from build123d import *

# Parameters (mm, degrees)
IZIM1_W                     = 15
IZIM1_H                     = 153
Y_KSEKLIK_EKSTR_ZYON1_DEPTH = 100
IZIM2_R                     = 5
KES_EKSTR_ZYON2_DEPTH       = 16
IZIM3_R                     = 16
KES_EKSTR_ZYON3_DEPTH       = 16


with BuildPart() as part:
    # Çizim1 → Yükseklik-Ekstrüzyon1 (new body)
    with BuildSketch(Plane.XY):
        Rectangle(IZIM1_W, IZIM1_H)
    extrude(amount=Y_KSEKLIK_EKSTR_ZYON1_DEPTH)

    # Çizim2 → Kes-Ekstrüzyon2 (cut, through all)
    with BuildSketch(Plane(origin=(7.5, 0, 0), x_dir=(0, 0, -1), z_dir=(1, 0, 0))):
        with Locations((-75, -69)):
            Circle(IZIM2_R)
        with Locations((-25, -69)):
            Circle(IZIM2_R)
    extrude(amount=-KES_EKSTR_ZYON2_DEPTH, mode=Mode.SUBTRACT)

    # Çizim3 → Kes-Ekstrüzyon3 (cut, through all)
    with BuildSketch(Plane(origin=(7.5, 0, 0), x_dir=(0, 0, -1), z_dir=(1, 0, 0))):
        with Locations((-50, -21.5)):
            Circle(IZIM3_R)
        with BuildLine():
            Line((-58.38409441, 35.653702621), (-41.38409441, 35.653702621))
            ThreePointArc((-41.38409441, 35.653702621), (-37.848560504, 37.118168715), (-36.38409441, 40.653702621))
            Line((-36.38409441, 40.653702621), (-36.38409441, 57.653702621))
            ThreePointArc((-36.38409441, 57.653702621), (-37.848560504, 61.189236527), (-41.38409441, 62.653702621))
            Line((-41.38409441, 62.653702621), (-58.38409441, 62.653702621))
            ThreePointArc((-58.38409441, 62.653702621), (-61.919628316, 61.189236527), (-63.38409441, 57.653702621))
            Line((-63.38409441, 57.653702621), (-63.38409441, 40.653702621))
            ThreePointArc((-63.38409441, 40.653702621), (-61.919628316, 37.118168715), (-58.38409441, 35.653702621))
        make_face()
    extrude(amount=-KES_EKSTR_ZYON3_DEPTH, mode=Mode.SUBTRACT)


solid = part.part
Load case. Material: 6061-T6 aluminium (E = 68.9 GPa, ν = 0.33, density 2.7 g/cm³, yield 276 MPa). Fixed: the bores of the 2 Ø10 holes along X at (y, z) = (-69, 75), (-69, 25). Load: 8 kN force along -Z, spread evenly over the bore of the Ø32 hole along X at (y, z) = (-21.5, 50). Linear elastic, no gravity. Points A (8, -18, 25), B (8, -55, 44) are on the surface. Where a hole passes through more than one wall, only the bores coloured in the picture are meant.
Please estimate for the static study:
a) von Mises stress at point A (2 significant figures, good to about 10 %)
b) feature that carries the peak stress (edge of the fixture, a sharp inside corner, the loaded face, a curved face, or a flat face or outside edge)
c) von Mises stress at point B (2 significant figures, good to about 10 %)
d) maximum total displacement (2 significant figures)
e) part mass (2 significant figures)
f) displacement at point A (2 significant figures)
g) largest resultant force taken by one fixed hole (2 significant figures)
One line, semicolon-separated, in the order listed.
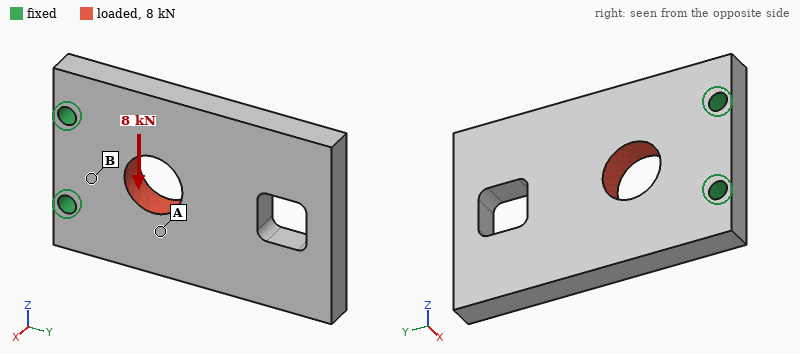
9.6 MPa; edge of the fixture; 20 MPa; 59 µm; 550 g; 29 µm; 7.4 kN
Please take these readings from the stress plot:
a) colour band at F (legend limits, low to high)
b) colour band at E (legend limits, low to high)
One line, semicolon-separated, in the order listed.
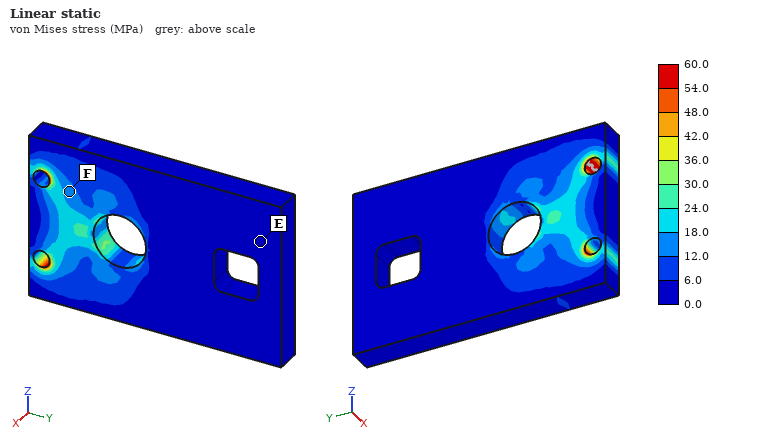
12.0 to 18.0 MPa; 0.0 to 6.0 MPa
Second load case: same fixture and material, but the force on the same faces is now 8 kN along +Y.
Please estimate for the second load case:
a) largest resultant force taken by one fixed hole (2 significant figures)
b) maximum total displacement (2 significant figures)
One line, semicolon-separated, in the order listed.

4.0 kN; 8.5 µm
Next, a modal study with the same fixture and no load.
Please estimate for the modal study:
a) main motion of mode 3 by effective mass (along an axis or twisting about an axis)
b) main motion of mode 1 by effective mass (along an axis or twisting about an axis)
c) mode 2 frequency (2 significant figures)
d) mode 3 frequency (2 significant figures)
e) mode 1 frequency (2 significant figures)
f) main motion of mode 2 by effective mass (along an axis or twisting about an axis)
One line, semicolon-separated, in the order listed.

along Z; along X; 1600 Hz; 2200 Hz; 550 Hz; twisting about Y
